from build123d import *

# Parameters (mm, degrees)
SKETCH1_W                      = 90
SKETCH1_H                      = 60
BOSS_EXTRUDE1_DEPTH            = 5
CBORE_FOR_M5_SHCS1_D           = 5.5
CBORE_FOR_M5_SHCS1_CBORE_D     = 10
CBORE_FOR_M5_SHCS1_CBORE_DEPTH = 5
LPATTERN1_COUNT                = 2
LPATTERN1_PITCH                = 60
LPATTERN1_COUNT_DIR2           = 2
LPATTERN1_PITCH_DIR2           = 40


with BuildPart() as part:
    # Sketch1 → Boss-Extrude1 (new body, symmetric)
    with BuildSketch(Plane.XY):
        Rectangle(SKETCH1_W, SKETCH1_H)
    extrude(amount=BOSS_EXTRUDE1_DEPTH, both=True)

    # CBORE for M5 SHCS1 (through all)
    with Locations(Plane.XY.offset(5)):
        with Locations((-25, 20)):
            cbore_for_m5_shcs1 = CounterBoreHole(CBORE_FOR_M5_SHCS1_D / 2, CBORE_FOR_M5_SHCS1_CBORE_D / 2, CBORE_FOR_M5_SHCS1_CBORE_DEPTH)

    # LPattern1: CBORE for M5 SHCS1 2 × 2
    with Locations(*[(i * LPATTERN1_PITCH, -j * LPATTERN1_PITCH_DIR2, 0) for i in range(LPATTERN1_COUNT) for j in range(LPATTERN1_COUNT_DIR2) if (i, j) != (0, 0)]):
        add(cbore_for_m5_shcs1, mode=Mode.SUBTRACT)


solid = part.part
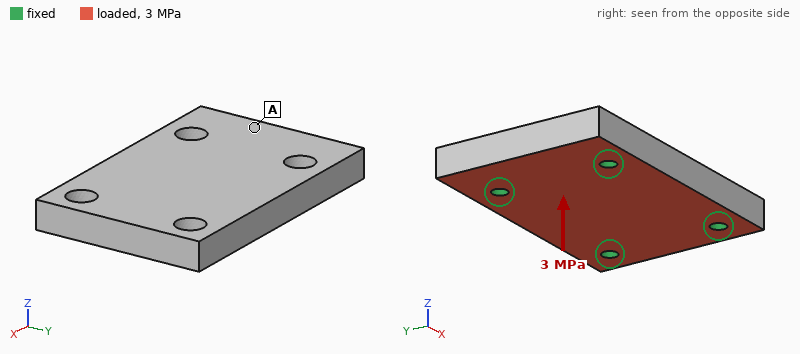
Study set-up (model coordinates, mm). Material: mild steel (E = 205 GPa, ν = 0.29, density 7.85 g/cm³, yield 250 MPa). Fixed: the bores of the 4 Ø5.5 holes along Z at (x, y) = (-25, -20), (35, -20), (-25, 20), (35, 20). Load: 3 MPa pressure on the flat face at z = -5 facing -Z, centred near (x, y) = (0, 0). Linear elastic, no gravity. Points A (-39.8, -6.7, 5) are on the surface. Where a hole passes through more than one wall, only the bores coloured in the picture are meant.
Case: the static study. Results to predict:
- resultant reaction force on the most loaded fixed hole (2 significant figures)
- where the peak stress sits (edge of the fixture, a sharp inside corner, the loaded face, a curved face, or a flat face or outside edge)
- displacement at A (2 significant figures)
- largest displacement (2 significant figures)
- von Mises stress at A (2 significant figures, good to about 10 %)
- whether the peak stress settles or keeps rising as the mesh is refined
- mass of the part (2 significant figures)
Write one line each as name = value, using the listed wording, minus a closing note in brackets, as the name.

resultant reaction force on the most loaded fixed hole = 4.8 kN
where the peak stress sits = edge of the fixture
displacement at A = 5.5 µm
largest displacement = 14 µm
von Mises stress at A = 16 MPa
whether the peak stress settles or keeps rising as the mesh is refined = keeps rising
mass of the part = 410 g
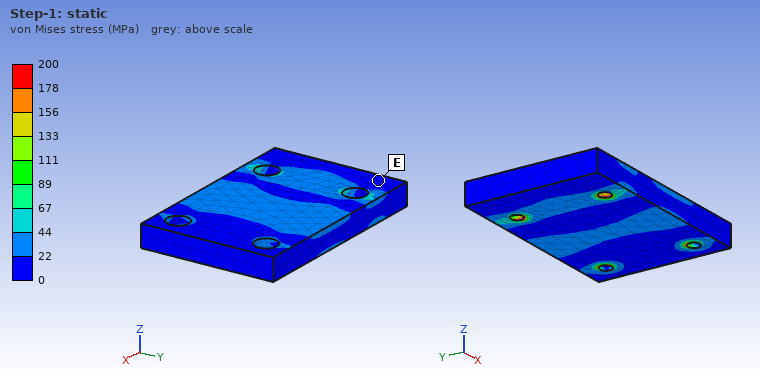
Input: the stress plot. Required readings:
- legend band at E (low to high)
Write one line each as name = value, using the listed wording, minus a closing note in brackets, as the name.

legend band at E = 0 to 22 MPa
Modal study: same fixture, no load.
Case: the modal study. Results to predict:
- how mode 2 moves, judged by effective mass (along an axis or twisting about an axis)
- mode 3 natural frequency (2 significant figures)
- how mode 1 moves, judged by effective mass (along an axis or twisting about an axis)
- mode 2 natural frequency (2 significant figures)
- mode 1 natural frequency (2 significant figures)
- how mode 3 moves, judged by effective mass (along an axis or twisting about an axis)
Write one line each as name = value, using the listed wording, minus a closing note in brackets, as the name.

how mode 2 moves, judged by effective mass = along Z
mode 3 natural frequency = 12 kHz
how mode 1 moves, judged by effective mass = along Z
mode 2 natural frequency = 11 kHz
mode 1 natural frequency = 8500 Hz
how mode 3 moves, judged by effective mass = twisting about X
